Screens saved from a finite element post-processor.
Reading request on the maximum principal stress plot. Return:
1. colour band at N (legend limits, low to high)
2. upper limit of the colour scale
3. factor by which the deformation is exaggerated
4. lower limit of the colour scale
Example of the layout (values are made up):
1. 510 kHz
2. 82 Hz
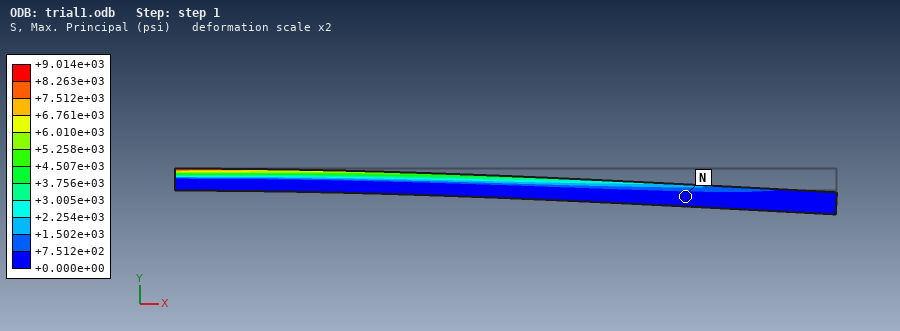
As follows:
1. +0.000e+00 to +7.512e+02 psi
2. +9.014e+03 psi
3. 2
4. +0.000e+00 psi
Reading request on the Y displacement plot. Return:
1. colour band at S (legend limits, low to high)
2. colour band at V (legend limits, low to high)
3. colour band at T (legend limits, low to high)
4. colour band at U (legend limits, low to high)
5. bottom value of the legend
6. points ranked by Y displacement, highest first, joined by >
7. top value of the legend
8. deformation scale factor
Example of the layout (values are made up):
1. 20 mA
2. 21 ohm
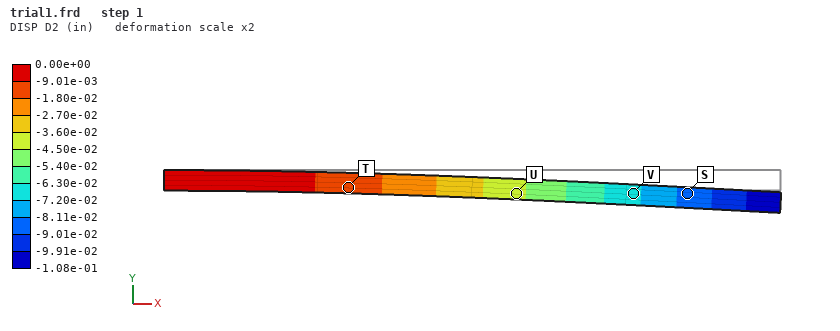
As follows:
1. -9.01e-02 to -8.11e-02 in
2. -7.20e-02 to -6.30e-02 in
3. -1.80e-02 to -9.01e-03 in
4. -4.50e-02 to -3.60e-02 in
5. -1.08e-01 in
6. T > U > V > S
7. 0.00e+00 in
8. 2
